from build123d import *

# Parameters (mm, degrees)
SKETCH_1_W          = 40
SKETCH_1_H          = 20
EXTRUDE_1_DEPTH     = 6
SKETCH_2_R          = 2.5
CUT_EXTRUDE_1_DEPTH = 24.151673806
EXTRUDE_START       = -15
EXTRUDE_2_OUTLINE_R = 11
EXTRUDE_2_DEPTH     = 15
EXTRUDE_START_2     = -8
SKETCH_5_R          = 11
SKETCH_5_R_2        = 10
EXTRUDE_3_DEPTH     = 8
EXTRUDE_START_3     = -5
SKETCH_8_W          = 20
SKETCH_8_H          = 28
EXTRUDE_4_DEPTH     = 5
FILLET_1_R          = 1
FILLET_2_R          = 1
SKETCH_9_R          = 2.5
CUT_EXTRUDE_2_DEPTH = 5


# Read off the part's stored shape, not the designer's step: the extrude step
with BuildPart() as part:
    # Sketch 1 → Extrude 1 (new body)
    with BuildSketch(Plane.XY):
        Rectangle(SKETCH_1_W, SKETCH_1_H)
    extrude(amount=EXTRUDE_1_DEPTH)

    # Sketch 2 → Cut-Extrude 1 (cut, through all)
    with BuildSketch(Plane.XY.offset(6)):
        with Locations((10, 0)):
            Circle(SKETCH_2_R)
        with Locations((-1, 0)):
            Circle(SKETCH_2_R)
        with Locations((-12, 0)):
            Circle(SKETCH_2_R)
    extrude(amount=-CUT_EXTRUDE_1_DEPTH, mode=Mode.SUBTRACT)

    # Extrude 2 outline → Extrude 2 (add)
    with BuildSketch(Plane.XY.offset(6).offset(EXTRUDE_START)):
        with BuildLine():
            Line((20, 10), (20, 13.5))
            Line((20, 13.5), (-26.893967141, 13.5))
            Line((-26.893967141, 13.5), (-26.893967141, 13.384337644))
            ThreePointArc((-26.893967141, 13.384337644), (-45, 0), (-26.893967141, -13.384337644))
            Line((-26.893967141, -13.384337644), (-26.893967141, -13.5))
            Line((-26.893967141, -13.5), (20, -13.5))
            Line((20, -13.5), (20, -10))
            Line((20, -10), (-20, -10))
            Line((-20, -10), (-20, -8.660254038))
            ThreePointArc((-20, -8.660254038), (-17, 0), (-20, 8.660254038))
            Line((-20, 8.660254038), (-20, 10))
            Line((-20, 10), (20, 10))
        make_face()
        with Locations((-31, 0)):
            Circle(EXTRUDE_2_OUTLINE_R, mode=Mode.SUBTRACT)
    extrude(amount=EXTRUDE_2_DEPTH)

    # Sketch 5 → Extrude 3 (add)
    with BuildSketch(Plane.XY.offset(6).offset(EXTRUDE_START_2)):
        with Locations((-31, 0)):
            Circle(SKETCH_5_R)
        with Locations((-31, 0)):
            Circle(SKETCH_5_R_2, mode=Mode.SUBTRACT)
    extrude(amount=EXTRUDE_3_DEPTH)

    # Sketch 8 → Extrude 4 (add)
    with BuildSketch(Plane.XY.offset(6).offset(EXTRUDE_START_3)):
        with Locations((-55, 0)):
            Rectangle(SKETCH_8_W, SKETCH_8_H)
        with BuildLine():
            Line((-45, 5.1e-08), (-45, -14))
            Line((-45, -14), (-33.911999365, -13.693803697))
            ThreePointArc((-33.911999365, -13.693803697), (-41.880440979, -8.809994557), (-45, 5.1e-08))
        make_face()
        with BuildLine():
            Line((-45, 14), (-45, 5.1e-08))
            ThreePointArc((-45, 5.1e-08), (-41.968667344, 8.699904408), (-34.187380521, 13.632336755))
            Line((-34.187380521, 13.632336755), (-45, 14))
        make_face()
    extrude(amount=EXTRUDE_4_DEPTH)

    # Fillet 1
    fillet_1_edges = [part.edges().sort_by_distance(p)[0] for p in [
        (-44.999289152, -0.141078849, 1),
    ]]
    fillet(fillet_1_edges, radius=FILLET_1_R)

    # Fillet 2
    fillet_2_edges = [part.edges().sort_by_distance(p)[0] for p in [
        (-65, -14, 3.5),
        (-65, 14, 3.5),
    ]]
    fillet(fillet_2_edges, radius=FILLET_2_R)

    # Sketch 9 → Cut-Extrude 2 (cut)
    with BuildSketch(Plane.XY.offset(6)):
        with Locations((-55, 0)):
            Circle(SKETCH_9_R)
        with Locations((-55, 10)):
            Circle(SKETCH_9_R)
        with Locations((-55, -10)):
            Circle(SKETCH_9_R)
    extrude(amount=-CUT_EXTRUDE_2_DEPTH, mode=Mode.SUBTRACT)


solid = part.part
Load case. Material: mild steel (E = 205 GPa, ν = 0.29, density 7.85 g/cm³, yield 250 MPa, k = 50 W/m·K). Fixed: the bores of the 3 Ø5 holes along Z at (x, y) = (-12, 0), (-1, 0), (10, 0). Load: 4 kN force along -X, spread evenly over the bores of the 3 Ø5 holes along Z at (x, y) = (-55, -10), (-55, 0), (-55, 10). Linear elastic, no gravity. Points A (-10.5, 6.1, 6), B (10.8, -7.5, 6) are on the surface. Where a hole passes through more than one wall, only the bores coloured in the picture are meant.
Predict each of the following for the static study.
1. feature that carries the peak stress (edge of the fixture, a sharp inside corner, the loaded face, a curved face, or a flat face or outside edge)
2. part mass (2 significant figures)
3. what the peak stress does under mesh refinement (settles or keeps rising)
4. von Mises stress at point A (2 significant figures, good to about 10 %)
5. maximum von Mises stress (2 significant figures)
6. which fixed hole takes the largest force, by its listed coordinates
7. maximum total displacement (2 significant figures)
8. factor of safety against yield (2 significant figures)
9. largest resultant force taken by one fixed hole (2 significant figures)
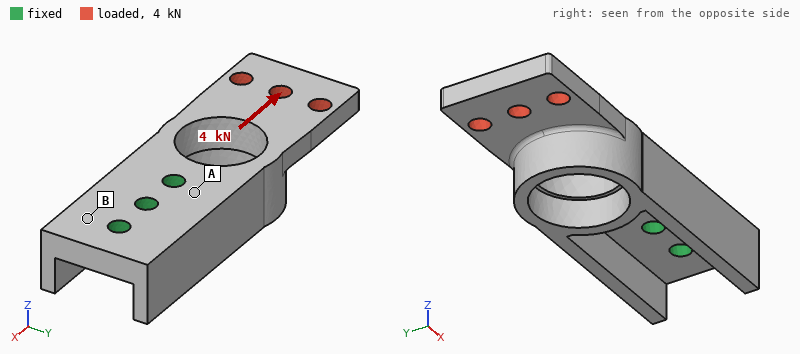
a curved face
120 g
settles
32 MPa
200 MPa
(-12, 0)
49 µm
1.3
2.0 kN
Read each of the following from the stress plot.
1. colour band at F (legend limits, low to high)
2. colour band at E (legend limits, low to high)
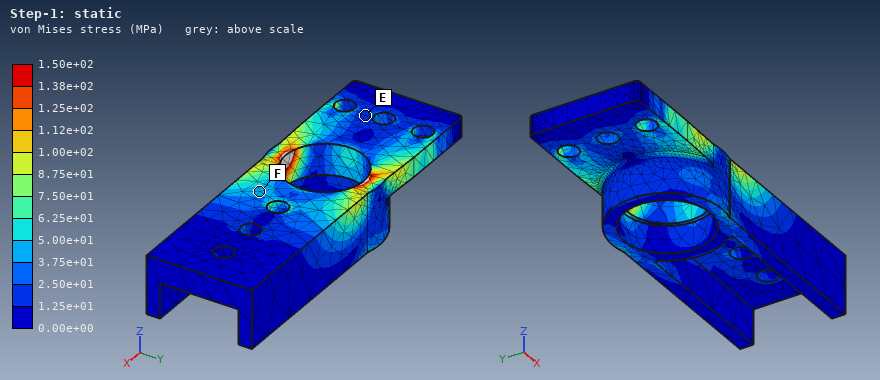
3.75e+01 to 5.00e+01 MPa
1.25e+01 to 2.50e+01 MPa
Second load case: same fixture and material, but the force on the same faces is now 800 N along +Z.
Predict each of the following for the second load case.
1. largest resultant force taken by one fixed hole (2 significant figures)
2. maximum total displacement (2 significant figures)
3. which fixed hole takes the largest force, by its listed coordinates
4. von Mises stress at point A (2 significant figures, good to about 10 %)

2.0 kN
0.13 mm
(-12, 0)
42 MPa
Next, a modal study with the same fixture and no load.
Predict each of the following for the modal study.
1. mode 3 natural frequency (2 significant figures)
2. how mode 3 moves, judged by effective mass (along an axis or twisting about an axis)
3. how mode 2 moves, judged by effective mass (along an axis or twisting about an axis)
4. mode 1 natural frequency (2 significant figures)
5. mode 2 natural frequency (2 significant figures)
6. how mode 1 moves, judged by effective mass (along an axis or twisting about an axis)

6200 Hz
twisting about X
along Y
3000 Hz
4700 Hz
along Z
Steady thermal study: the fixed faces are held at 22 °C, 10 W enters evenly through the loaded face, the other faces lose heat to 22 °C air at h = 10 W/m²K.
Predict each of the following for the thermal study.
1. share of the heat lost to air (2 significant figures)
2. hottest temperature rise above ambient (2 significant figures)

16 %
65 K
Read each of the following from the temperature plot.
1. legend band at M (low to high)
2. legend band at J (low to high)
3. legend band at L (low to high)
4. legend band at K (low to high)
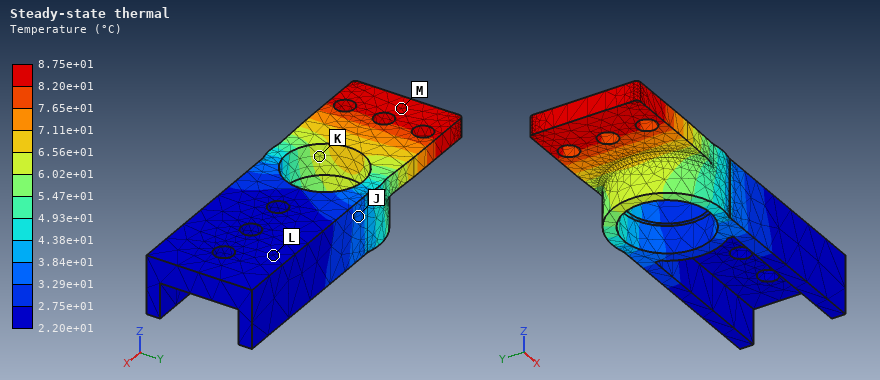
8.20e+01 to 8.75e+01 °C
3.29e+01 to 3.84e+01 °C
2.20e+01 to 2.75e+01 °C
6.02e+01 to 6.56e+01 °C
